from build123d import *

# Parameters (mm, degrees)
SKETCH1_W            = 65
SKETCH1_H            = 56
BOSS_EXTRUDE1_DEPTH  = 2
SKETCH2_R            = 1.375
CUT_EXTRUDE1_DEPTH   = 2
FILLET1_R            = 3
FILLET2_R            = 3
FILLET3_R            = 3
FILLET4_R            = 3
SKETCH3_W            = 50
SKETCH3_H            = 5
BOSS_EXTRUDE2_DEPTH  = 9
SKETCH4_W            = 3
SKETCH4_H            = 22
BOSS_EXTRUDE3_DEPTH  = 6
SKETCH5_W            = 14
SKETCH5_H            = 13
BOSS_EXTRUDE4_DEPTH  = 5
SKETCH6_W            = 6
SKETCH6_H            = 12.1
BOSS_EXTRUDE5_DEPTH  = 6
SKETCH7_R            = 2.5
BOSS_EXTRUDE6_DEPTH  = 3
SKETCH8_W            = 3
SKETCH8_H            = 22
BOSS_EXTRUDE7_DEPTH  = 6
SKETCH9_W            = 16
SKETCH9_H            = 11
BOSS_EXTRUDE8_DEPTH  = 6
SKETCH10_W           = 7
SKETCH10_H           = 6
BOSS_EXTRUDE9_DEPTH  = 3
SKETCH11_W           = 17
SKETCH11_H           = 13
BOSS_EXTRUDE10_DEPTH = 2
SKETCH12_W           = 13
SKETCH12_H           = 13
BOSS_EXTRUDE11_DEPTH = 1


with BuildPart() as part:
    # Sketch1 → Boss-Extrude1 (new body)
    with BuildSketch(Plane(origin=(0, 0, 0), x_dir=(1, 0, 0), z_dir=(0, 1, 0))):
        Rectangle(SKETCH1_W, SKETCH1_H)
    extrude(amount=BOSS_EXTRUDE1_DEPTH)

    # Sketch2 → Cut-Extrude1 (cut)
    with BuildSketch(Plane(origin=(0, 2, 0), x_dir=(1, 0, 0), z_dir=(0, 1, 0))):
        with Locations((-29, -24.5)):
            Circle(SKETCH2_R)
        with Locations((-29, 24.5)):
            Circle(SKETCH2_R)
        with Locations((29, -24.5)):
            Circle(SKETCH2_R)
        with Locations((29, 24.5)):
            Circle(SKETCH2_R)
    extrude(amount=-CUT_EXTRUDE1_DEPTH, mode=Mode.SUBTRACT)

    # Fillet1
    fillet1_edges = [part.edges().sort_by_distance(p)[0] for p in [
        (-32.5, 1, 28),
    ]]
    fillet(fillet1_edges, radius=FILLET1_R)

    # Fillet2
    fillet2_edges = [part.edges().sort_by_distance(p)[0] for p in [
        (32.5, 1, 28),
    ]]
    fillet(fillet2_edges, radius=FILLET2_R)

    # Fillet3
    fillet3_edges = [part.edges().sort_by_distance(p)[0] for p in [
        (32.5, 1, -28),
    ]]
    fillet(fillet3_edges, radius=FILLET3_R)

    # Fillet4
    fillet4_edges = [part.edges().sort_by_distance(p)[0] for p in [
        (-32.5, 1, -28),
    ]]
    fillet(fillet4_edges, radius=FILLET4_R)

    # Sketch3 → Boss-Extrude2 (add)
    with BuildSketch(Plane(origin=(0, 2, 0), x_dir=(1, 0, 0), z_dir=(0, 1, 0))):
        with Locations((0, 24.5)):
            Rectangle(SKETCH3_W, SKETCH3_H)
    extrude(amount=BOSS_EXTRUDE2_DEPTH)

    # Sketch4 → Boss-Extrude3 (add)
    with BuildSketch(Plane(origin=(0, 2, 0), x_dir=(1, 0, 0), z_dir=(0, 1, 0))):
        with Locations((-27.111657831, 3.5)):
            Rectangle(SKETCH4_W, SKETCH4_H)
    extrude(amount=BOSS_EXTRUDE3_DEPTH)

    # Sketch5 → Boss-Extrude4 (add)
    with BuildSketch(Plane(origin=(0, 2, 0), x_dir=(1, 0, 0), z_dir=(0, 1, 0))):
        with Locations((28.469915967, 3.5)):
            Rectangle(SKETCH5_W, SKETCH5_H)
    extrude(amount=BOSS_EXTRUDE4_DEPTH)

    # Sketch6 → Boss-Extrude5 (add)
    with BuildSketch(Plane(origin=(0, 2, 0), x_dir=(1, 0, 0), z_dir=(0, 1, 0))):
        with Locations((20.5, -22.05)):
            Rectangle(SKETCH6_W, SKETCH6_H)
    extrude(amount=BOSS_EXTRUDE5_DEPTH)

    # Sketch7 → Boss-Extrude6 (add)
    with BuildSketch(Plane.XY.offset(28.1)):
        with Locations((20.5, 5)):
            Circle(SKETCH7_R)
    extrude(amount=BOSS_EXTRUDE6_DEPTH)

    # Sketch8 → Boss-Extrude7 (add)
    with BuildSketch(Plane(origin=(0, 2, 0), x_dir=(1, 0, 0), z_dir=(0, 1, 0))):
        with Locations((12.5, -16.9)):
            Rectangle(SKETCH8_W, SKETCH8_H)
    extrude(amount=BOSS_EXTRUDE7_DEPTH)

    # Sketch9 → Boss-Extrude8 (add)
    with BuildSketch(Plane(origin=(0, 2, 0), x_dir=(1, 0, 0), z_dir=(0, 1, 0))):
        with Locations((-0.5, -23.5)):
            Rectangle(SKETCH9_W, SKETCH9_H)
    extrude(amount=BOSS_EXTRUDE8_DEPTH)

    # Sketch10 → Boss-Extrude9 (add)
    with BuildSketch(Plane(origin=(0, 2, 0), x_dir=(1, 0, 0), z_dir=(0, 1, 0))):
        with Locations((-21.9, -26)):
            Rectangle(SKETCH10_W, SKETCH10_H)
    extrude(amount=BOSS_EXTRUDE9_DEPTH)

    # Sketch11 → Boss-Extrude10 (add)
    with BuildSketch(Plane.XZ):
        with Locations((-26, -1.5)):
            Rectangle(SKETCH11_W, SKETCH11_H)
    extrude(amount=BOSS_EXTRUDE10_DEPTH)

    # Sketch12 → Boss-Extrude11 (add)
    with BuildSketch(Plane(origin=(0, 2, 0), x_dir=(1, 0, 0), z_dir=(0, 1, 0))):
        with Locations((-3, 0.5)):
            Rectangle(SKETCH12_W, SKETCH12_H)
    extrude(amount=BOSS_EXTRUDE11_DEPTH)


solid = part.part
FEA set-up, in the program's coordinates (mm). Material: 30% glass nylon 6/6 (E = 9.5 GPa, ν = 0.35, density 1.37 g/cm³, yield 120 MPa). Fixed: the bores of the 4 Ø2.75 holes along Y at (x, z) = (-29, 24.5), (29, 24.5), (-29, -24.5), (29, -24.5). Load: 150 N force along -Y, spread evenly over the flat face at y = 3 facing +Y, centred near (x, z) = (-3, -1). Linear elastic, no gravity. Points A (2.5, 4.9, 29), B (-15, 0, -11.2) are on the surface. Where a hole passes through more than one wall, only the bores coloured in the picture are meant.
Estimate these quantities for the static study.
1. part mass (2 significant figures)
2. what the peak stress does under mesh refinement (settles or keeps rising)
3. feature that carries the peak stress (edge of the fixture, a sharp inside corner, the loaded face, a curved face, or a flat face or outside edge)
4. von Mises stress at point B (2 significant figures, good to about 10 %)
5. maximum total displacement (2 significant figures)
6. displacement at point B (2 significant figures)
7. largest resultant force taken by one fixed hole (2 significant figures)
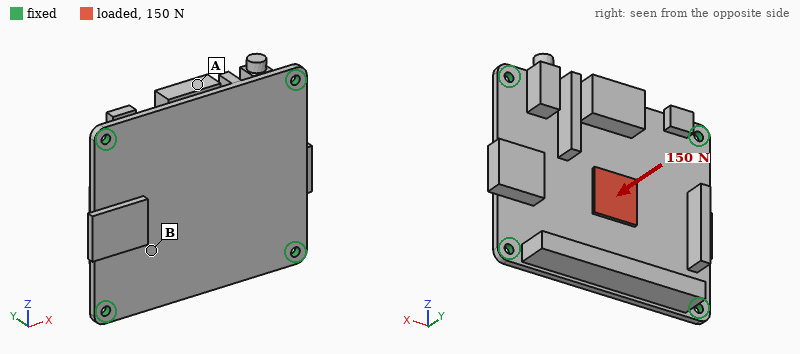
18 g
keeps rising
edge of the fixture
17 MPa
0.43 mm
0.23 mm
65 N
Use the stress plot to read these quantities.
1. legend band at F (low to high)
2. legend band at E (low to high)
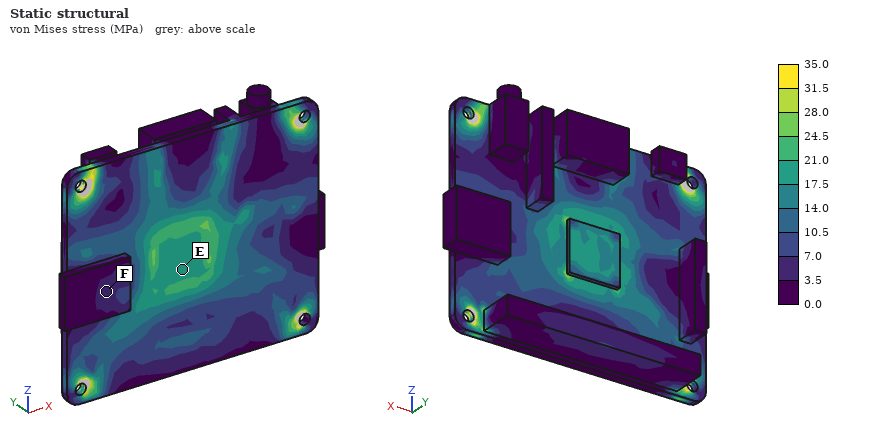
3.5 to 7.0 MPa
17.5 to 21.0 MPa
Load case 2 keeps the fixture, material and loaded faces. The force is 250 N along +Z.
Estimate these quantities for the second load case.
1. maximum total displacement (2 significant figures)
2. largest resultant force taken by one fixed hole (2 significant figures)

49 µm
80 N
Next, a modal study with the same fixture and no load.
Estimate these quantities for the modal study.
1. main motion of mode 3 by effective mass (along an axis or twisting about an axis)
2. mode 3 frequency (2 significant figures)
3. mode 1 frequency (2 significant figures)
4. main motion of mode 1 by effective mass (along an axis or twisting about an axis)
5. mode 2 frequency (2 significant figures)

twisting about Z
2300 Hz
1300 Hz
along Y
1900 Hz
